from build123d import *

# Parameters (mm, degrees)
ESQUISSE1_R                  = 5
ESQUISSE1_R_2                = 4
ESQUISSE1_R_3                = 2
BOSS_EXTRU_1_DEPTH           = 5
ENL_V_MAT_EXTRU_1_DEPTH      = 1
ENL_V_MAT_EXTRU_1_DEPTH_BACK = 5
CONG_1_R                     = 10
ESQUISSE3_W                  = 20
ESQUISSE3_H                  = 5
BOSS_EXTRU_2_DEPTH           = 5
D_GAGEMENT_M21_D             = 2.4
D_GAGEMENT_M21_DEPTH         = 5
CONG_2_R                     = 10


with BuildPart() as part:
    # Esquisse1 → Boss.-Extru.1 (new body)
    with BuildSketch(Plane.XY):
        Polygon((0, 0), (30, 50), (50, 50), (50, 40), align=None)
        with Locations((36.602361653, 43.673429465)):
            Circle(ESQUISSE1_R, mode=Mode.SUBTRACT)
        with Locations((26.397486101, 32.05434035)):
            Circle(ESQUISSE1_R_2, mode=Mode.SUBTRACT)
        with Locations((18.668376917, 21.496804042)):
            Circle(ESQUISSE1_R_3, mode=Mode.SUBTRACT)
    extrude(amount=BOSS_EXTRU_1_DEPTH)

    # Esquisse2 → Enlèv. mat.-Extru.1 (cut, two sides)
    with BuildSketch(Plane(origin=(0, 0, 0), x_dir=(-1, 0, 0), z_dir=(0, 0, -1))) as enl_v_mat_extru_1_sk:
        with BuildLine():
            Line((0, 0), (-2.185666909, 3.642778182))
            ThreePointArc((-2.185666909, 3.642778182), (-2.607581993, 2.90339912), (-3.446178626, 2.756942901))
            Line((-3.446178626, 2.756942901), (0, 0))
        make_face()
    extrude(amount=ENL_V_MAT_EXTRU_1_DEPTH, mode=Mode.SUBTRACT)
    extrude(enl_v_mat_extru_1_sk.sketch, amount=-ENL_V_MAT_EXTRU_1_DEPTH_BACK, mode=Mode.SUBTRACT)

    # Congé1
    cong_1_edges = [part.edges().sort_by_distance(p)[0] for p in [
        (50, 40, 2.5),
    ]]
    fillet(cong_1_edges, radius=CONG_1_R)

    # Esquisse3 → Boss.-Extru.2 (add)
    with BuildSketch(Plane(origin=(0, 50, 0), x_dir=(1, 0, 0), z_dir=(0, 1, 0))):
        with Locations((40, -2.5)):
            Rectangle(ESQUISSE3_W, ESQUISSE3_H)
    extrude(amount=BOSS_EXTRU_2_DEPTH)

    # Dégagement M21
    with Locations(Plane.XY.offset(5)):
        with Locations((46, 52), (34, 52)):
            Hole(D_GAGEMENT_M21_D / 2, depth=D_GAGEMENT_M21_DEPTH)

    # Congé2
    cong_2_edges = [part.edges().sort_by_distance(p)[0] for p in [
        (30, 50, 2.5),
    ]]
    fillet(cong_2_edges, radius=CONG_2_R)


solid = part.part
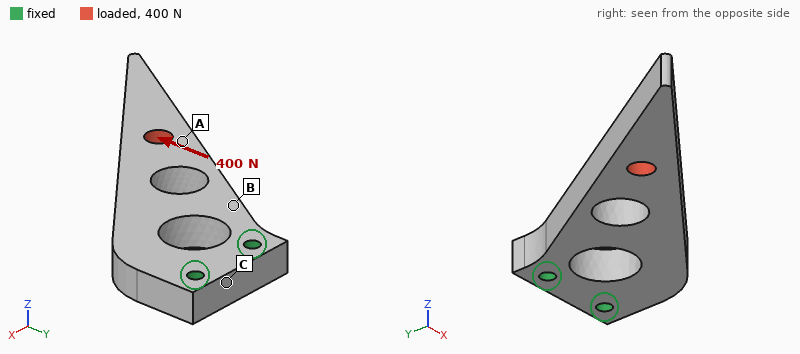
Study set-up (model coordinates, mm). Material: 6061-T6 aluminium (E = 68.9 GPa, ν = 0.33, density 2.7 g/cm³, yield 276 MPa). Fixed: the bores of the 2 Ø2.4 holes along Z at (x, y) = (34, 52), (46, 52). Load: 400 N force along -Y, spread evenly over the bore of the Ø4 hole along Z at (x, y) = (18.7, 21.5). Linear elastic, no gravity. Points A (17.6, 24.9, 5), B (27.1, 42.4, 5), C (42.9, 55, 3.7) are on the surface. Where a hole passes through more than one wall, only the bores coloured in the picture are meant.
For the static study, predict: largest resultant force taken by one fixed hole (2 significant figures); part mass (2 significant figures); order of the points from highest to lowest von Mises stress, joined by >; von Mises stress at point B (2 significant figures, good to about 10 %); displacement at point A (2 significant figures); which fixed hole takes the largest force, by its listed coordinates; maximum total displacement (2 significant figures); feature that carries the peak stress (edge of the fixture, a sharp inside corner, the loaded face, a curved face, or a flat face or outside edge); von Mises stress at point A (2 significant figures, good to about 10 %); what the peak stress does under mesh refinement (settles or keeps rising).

810 N
9.4 g
B > A > C
26 MPa
39 µm
(34, 52)
75 µm
edge of the fixture
15 MPa
keeps rising
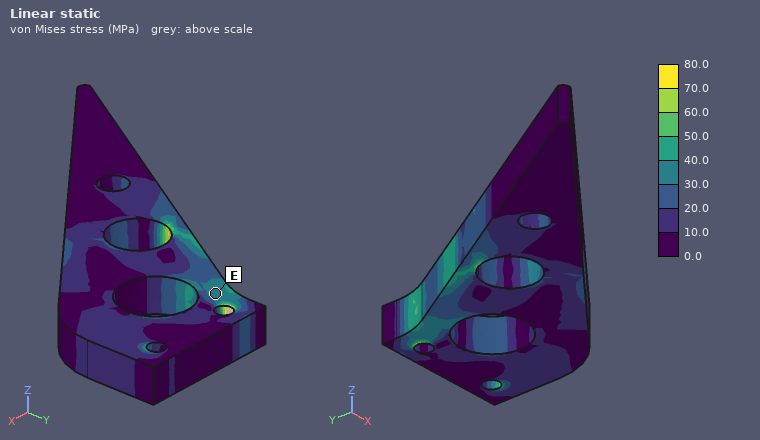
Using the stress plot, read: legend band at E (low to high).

30.0 to 40.0 MPa
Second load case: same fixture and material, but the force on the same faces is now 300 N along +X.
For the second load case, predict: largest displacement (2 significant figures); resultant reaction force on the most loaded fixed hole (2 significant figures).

71 µm
660 N
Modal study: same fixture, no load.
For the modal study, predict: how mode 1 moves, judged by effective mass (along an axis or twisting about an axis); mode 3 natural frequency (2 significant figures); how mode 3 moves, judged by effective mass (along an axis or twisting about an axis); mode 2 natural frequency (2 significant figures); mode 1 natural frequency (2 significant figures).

along Z
7000 Hz
along Z
5400 Hz
1600 Hz
